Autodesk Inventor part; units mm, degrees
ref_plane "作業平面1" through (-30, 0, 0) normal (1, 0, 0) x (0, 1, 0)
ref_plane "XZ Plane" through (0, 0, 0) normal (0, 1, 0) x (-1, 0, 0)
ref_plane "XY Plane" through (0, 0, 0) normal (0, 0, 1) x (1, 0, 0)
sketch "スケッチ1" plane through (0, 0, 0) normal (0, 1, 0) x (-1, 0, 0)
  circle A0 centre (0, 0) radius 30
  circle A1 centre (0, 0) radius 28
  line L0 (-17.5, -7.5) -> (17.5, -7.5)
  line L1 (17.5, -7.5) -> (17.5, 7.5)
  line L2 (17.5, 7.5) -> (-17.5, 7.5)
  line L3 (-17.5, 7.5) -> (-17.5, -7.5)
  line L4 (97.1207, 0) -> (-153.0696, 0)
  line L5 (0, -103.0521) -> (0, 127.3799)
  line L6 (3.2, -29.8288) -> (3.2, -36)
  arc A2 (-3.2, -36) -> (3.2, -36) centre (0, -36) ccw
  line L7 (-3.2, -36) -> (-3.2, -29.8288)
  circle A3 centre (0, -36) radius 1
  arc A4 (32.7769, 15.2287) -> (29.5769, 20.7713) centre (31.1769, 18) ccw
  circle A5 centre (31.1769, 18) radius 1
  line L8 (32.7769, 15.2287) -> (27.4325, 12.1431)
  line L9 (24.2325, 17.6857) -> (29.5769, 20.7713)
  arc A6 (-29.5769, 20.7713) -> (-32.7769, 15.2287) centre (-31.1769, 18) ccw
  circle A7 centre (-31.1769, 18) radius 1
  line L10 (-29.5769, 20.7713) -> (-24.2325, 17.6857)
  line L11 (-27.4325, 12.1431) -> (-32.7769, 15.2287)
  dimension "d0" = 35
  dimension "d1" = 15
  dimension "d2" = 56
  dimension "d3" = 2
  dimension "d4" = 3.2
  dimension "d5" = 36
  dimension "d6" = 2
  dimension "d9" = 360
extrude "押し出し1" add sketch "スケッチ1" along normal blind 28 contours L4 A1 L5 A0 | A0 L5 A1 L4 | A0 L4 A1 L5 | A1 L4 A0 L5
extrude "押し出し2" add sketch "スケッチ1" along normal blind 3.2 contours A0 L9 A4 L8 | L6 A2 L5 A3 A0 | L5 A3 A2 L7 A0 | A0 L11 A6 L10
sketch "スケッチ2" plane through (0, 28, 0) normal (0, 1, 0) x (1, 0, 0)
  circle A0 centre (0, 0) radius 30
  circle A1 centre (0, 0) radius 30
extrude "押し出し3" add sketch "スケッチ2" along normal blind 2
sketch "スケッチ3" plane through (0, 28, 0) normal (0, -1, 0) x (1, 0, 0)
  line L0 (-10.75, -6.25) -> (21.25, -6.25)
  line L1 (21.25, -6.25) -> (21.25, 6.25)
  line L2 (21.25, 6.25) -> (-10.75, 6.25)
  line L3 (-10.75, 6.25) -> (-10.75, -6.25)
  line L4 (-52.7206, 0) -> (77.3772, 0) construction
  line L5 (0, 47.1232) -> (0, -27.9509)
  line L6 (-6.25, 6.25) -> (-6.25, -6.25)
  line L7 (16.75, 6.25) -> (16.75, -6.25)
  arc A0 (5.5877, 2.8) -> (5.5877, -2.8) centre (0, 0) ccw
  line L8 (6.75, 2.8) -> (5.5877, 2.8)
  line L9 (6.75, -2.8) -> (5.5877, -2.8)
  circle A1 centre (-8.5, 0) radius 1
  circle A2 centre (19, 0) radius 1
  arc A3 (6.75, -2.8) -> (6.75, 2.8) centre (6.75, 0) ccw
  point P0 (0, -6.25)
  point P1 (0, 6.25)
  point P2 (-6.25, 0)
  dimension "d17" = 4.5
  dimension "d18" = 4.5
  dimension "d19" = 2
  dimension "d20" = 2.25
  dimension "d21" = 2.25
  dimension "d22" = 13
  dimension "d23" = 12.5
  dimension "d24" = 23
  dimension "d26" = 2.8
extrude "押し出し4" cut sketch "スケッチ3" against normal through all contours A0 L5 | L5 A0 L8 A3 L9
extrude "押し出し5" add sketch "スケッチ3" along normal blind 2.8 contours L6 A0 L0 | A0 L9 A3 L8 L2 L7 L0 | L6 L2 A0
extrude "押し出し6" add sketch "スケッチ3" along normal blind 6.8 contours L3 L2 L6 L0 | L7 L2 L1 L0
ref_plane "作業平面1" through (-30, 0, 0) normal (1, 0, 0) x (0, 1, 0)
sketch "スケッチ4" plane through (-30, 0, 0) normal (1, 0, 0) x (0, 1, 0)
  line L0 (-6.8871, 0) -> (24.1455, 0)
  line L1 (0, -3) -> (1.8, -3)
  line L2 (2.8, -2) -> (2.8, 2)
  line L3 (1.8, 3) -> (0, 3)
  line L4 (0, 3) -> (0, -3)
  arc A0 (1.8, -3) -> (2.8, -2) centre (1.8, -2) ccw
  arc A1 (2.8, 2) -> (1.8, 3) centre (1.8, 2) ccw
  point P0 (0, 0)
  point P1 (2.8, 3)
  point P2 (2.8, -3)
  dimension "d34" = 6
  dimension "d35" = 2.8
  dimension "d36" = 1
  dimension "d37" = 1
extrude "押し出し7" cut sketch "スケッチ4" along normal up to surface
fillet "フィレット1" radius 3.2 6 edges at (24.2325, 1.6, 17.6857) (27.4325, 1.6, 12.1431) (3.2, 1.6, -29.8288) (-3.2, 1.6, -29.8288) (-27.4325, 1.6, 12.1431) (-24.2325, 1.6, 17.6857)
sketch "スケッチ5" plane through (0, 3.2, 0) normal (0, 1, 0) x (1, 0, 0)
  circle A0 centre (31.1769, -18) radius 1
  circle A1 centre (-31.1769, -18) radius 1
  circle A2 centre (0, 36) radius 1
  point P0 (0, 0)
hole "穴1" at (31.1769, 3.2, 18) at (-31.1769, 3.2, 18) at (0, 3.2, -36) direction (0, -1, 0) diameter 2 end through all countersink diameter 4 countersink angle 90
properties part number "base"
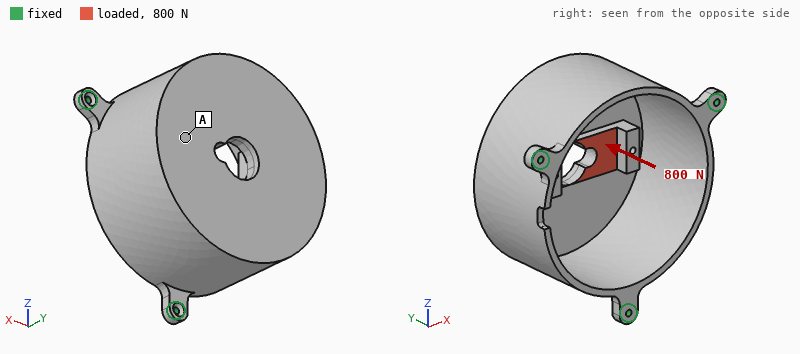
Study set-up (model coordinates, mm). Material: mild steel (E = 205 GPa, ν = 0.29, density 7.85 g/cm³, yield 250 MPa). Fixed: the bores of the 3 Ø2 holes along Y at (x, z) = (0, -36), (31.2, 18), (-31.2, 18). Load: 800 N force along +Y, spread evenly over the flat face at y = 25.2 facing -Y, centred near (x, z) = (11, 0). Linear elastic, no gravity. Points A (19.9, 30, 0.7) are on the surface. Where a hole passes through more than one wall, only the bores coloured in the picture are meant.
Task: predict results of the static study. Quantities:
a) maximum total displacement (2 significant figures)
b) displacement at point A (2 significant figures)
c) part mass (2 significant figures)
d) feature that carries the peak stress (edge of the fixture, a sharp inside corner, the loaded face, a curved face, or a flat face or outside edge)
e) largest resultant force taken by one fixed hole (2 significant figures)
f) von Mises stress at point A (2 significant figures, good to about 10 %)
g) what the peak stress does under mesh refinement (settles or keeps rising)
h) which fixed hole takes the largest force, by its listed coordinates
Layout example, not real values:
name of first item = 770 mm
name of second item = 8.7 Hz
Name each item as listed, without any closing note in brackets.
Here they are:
maximum total displacement = 61 µm
displacement at point A = 31 µm
part mass = 140 g
feature that carries the peak stress = a sharp inside corner
largest resultant force taken by one fixed hole = 440 N
von Mises stress at point A = 24 MPa
what the peak stress does under mesh refinement = keeps rising
which fixed hole takes the largest force, by its listed coordinates = (31.2, 18)
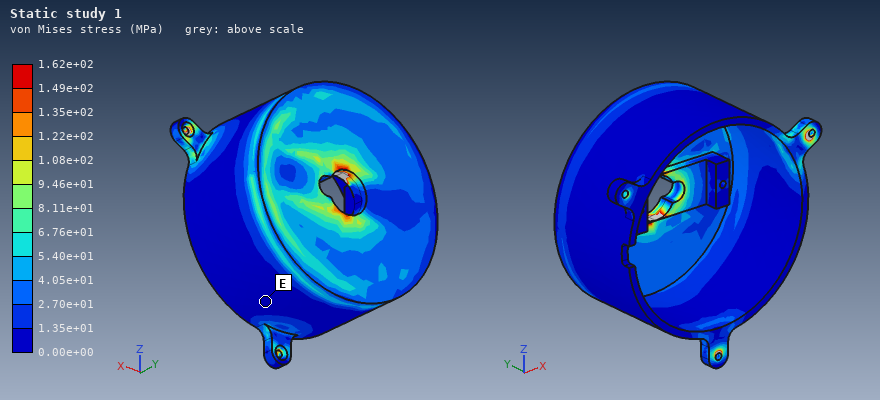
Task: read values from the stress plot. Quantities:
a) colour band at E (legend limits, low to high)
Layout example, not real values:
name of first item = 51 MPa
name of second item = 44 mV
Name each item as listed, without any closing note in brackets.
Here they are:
colour band at E = 0.00e+00 to 1.35e+01 MPa
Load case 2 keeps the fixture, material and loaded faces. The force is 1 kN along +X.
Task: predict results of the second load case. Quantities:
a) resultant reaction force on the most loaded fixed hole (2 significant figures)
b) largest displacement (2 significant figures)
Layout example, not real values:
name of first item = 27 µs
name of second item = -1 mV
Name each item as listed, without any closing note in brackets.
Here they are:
resultant reaction force on the most loaded fixed hole = 540 N
largest displacement = 28 µm
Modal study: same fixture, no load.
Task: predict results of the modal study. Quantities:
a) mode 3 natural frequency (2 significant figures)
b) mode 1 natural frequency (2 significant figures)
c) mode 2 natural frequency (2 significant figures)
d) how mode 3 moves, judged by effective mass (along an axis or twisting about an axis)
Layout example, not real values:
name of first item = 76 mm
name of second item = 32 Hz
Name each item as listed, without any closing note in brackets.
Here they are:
mode 3 natural frequency = 3900 Hz
mode 1 natural frequency = 3500 Hz
mode 2 natural frequency = 3500 Hz
how mode 3 moves, judged by effective mass = along Y
